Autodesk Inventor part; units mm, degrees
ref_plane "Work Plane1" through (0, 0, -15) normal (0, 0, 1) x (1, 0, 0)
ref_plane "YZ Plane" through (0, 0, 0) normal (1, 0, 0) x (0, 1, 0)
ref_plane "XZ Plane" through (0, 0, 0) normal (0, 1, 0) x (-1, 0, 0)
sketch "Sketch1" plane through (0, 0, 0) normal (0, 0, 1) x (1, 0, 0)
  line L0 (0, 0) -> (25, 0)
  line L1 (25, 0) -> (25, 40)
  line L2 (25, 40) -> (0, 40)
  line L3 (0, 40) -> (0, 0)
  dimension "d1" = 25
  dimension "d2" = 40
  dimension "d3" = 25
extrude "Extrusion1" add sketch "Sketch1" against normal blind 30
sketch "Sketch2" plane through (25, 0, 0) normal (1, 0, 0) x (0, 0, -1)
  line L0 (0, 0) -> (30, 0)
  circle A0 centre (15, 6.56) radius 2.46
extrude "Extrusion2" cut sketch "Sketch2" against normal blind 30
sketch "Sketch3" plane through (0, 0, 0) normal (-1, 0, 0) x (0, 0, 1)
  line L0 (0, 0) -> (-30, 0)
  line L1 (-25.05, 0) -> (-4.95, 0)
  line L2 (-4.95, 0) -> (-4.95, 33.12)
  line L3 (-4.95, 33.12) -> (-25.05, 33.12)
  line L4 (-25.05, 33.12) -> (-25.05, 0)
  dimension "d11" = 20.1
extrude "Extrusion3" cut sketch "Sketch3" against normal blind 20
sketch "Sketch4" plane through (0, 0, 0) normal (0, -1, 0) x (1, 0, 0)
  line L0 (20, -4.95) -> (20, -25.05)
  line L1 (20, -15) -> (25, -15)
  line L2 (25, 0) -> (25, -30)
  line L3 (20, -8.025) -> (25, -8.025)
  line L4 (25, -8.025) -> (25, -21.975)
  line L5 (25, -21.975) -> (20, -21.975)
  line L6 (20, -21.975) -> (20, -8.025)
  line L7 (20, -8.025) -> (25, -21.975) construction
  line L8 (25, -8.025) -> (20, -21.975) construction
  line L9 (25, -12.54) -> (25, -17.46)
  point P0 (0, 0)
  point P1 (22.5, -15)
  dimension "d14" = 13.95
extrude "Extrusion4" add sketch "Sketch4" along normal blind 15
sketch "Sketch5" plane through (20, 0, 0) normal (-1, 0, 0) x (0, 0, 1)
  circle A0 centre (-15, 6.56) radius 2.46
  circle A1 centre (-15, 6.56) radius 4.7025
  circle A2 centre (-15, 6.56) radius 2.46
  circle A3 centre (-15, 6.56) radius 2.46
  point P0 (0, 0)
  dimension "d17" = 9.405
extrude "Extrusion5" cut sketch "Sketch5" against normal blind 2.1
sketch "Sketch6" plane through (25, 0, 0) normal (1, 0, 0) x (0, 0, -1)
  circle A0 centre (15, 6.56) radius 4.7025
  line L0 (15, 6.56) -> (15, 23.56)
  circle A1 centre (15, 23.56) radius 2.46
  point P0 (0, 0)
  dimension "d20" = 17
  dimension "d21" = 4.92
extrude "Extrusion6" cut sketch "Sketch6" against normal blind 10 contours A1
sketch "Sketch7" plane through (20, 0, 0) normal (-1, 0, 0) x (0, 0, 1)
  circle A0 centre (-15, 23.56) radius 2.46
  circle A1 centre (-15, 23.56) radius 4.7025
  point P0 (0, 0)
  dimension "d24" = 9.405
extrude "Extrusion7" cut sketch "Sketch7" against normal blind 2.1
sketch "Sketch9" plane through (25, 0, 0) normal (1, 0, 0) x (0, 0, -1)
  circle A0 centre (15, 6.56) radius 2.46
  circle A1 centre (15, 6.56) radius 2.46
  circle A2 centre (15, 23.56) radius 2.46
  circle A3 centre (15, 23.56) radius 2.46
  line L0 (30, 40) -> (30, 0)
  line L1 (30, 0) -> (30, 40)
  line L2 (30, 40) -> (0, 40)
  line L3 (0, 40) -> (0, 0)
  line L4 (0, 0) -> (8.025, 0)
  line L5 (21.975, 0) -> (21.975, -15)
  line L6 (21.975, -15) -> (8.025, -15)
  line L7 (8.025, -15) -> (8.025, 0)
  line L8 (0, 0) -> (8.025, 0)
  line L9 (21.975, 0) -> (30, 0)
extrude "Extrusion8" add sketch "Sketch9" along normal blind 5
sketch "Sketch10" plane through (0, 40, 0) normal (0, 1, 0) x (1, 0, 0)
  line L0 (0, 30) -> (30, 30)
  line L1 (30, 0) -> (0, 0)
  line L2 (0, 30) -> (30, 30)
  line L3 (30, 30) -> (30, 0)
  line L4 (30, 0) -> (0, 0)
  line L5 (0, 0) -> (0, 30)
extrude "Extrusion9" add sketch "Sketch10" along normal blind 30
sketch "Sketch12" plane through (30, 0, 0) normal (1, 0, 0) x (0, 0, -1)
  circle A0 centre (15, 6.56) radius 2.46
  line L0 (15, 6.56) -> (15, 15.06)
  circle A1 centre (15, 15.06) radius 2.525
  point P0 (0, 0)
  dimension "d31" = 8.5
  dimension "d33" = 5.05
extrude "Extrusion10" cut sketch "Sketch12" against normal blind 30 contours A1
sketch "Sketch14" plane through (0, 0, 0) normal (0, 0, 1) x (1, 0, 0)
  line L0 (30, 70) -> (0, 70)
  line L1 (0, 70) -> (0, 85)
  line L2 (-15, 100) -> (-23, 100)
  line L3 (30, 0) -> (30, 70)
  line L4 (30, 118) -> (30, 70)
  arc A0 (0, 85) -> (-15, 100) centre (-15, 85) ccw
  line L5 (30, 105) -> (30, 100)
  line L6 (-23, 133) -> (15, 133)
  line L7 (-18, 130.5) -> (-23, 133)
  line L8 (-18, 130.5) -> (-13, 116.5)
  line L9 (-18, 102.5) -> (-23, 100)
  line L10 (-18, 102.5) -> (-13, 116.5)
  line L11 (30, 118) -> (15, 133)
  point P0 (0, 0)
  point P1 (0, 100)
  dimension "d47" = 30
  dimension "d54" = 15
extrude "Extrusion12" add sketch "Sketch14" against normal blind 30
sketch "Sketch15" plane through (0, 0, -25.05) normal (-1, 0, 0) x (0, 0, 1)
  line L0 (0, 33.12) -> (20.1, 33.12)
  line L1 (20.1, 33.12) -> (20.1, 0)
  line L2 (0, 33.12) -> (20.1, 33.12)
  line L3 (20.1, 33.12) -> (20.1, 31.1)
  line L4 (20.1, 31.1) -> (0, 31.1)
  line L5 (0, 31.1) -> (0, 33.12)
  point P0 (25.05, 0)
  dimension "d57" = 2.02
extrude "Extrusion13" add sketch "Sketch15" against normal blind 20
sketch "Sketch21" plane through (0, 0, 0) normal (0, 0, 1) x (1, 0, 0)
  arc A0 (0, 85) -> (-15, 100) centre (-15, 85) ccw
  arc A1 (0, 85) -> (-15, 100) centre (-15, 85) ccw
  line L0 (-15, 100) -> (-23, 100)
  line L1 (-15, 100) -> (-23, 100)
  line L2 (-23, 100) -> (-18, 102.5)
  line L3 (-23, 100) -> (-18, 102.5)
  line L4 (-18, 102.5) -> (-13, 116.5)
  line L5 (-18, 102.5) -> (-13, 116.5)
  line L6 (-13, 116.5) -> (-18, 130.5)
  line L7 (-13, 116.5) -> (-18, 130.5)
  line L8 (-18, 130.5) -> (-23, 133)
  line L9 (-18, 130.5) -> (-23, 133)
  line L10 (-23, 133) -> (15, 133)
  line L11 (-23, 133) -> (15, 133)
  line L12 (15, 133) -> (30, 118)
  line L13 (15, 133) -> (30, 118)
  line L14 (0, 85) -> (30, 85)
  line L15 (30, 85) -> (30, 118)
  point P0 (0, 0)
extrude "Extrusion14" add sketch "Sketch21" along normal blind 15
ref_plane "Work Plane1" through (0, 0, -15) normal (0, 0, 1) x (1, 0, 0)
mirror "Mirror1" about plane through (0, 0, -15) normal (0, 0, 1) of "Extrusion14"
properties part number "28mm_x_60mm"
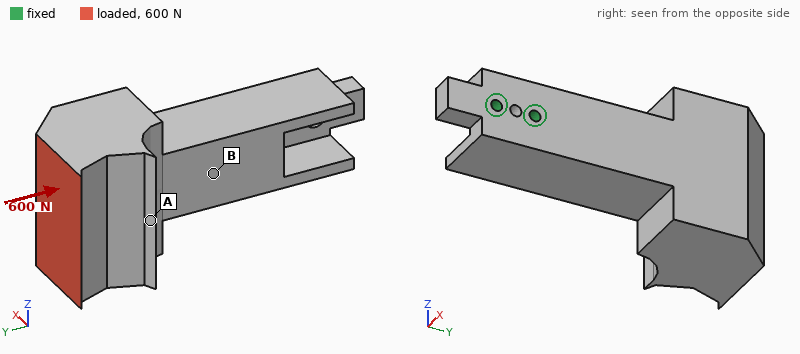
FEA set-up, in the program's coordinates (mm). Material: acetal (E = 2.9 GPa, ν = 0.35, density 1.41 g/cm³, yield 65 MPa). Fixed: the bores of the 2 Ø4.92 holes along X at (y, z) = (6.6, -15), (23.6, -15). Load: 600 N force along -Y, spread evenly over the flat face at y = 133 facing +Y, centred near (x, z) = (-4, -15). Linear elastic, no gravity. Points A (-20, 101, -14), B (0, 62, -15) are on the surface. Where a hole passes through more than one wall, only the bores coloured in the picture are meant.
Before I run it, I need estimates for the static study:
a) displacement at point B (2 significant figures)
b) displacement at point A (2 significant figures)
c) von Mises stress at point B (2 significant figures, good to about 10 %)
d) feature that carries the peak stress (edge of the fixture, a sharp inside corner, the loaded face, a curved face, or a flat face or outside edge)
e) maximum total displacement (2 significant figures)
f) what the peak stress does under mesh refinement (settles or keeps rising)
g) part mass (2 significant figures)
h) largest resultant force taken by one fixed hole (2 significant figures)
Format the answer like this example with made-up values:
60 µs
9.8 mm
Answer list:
0.48 mm
1.0 mm
3.1 MPa
edge of the fixture
1.4 mm
keeps rising
250 g
810 N
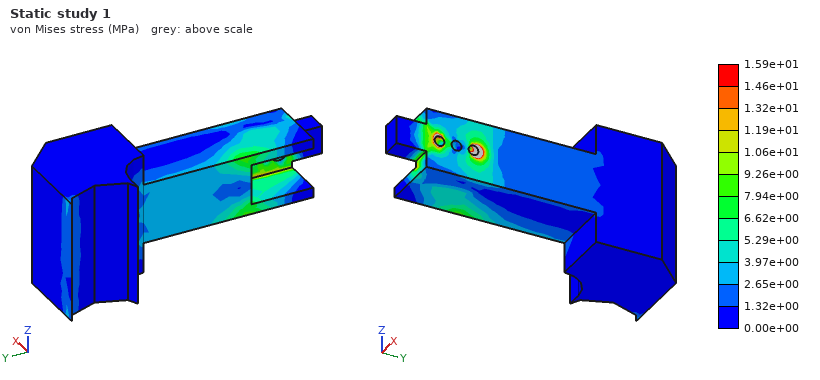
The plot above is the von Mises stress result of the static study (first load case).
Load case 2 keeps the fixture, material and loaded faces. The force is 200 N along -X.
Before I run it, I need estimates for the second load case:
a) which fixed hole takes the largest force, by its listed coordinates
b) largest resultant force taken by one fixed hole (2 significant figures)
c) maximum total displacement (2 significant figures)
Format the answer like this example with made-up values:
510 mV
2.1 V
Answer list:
(23.6, -15)
1.1 kN
1.8 mm
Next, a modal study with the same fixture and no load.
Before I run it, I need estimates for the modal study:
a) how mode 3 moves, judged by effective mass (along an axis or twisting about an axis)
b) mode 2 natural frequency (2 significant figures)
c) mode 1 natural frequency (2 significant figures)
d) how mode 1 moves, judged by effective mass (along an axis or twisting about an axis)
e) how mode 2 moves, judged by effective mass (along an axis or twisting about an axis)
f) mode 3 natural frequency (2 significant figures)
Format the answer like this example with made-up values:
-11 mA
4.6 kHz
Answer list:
twisting about Y
190 Hz
170 Hz
along X
along Z
440 Hz
